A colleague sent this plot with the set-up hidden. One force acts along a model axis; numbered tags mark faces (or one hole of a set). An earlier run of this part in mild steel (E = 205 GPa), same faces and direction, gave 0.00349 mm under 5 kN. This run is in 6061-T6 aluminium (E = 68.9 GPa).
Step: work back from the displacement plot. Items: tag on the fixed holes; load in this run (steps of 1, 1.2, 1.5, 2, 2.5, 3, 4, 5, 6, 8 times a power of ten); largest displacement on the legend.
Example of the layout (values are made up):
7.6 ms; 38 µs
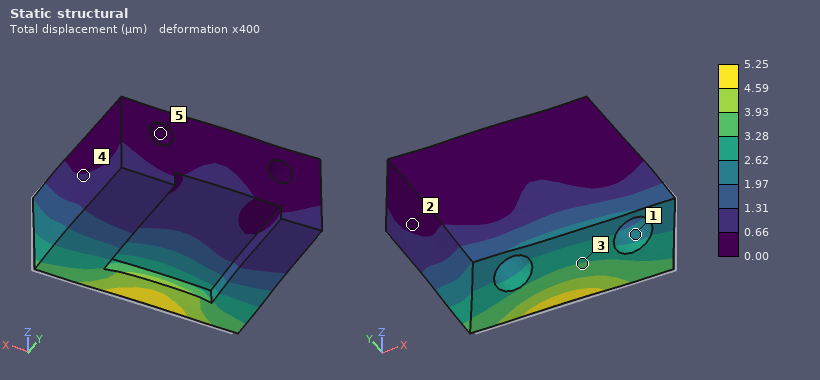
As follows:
5; 2.5 kN; 5.25 µm
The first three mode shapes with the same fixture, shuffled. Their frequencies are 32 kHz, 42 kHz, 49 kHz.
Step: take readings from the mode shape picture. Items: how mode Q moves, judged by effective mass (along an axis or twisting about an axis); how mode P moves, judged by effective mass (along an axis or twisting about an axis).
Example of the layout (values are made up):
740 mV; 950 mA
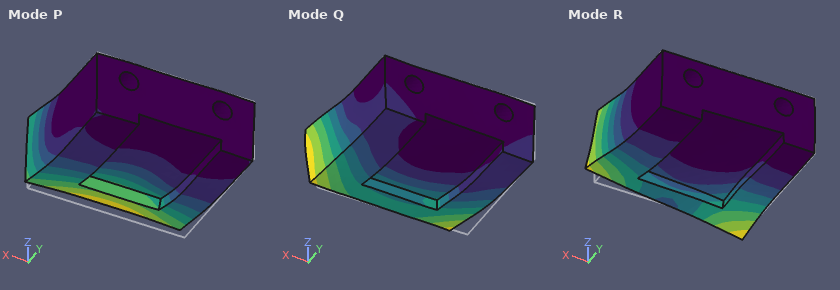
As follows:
along X; along Z
